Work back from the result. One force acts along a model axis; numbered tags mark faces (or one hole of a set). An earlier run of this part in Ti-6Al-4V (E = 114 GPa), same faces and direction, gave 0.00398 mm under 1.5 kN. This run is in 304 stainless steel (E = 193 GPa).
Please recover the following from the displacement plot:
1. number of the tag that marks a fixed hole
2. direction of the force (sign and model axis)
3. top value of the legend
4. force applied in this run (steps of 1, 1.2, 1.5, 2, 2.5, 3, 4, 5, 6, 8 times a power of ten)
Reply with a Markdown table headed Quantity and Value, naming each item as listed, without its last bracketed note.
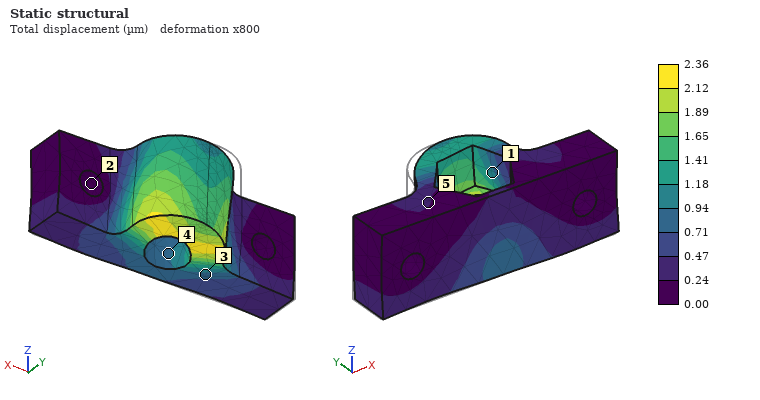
| Quantity | Value |
|---|---|
| number of the tag that marks a fixed hole | 2 |
| direction of the force | +X |
| top value of the legend | 2.36 µm |
| force applied in this run | 1.5 kN |
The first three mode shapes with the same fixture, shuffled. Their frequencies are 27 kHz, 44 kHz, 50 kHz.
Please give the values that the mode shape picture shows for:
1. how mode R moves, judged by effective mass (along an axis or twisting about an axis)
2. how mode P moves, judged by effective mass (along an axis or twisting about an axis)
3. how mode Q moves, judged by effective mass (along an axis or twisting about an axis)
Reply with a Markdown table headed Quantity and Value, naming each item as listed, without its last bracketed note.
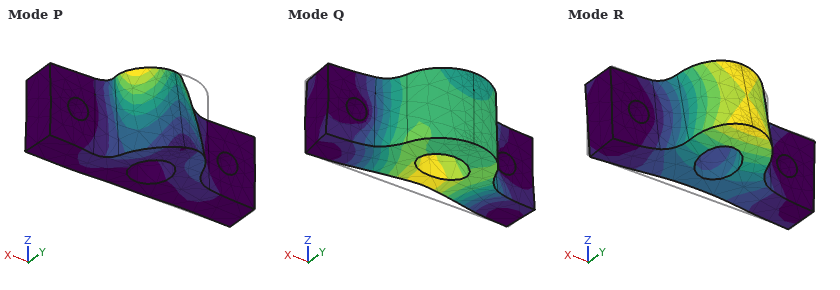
| Quantity | Value |
|---|---|
| how mode R moves, judged by effective mass | along Z |
| how mode P moves, judged by effective mass | along X |
| how mode Q moves, judged by effective mass | along Y |
